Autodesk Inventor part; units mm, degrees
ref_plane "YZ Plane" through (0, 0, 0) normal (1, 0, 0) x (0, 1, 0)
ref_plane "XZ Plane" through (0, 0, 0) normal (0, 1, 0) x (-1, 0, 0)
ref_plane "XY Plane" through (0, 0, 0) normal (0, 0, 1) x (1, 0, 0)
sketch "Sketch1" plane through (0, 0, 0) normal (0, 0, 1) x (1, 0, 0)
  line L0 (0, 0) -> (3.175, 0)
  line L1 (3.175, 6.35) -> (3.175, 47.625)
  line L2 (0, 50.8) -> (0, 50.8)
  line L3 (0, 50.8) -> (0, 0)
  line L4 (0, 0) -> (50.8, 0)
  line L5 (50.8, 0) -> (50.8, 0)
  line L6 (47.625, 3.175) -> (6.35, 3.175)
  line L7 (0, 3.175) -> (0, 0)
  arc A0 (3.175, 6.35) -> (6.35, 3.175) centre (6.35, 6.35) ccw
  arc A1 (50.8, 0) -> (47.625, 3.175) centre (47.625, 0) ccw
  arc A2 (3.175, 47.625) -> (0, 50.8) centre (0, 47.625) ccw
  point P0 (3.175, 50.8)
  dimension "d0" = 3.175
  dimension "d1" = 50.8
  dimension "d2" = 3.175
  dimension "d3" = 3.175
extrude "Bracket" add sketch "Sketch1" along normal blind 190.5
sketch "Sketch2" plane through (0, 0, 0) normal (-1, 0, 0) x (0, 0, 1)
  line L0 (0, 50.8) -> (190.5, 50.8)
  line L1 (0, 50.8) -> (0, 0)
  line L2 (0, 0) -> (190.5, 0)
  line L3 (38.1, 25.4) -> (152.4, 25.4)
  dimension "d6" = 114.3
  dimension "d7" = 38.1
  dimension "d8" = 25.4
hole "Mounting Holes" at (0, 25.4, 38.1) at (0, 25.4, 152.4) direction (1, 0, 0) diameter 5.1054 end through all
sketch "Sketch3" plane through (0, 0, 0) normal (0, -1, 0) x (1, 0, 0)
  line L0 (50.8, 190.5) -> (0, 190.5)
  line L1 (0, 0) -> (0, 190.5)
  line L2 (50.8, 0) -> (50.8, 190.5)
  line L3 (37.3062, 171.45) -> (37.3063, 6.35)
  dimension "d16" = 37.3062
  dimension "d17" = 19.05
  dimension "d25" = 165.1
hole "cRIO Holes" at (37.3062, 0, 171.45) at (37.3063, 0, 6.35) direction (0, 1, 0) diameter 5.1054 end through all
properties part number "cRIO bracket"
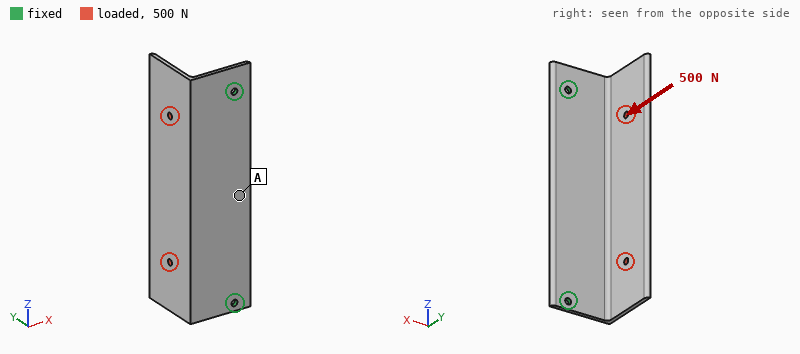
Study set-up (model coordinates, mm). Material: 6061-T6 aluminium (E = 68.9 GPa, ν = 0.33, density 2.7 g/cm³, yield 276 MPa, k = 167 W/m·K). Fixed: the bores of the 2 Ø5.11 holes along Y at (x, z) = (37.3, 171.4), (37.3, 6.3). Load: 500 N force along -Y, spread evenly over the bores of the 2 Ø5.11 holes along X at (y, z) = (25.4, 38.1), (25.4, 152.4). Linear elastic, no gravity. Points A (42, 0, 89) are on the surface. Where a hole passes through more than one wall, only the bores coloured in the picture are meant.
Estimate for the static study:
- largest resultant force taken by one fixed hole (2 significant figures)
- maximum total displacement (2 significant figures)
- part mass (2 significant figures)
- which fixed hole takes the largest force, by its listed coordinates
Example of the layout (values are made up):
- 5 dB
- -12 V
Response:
- 270 N
- 1.2 mm
- 160 g
- (37.3, 171.4)
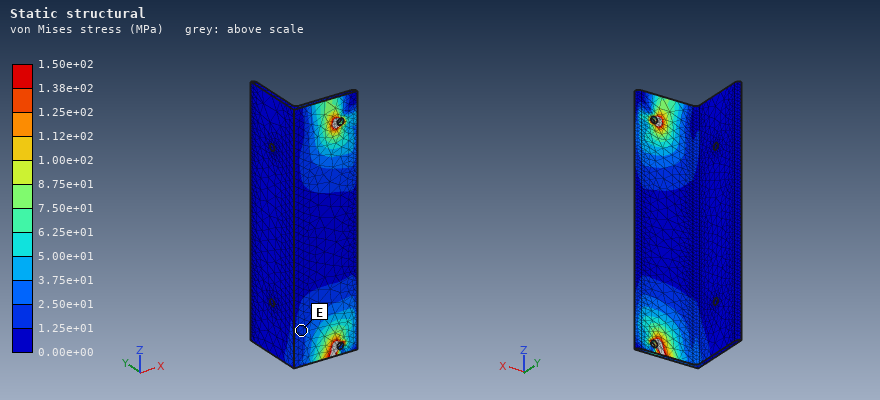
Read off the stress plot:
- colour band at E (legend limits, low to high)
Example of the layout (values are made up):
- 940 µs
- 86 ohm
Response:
- 1.25e+01 to 2.50e+01 MPa
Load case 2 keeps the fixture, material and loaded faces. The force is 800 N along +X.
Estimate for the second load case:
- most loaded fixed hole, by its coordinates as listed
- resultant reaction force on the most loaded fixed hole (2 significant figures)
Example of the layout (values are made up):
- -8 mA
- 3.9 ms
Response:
- (37.3, 171.4)
- 490 N
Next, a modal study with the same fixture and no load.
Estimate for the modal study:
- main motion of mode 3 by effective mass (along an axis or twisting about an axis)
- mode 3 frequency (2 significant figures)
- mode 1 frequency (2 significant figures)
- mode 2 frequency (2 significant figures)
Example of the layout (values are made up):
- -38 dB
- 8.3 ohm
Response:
- along Y
- 800 Hz
- 350 Hz
- 660 Hz
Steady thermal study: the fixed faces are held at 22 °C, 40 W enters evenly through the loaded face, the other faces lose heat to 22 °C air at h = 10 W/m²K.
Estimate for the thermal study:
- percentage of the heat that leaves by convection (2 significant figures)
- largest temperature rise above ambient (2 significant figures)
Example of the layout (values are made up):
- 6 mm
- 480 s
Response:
- 24 %
- 46 K
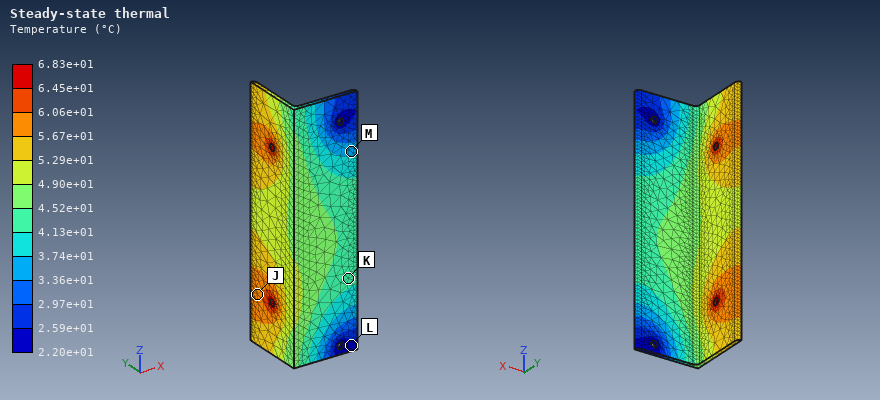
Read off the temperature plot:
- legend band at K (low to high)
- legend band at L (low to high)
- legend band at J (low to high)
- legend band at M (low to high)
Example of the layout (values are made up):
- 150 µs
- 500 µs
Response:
- 4.13e+01 to 4.52e+01 °C
- 2.20e+01 to 2.59e+01 °C
- 5.67e+01 to 6.06e+01 °C
- 3.36e+01 to 3.74e+01 °C
